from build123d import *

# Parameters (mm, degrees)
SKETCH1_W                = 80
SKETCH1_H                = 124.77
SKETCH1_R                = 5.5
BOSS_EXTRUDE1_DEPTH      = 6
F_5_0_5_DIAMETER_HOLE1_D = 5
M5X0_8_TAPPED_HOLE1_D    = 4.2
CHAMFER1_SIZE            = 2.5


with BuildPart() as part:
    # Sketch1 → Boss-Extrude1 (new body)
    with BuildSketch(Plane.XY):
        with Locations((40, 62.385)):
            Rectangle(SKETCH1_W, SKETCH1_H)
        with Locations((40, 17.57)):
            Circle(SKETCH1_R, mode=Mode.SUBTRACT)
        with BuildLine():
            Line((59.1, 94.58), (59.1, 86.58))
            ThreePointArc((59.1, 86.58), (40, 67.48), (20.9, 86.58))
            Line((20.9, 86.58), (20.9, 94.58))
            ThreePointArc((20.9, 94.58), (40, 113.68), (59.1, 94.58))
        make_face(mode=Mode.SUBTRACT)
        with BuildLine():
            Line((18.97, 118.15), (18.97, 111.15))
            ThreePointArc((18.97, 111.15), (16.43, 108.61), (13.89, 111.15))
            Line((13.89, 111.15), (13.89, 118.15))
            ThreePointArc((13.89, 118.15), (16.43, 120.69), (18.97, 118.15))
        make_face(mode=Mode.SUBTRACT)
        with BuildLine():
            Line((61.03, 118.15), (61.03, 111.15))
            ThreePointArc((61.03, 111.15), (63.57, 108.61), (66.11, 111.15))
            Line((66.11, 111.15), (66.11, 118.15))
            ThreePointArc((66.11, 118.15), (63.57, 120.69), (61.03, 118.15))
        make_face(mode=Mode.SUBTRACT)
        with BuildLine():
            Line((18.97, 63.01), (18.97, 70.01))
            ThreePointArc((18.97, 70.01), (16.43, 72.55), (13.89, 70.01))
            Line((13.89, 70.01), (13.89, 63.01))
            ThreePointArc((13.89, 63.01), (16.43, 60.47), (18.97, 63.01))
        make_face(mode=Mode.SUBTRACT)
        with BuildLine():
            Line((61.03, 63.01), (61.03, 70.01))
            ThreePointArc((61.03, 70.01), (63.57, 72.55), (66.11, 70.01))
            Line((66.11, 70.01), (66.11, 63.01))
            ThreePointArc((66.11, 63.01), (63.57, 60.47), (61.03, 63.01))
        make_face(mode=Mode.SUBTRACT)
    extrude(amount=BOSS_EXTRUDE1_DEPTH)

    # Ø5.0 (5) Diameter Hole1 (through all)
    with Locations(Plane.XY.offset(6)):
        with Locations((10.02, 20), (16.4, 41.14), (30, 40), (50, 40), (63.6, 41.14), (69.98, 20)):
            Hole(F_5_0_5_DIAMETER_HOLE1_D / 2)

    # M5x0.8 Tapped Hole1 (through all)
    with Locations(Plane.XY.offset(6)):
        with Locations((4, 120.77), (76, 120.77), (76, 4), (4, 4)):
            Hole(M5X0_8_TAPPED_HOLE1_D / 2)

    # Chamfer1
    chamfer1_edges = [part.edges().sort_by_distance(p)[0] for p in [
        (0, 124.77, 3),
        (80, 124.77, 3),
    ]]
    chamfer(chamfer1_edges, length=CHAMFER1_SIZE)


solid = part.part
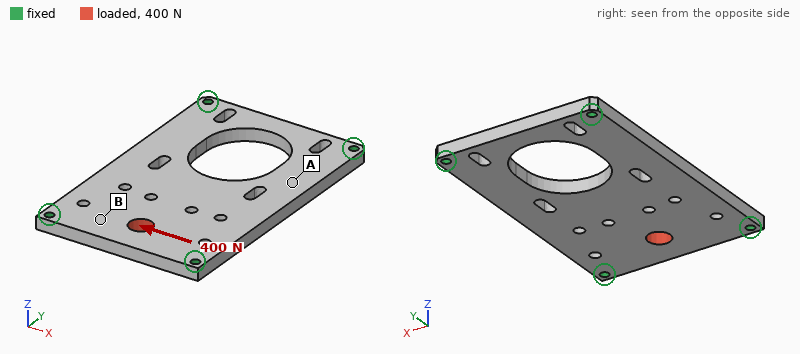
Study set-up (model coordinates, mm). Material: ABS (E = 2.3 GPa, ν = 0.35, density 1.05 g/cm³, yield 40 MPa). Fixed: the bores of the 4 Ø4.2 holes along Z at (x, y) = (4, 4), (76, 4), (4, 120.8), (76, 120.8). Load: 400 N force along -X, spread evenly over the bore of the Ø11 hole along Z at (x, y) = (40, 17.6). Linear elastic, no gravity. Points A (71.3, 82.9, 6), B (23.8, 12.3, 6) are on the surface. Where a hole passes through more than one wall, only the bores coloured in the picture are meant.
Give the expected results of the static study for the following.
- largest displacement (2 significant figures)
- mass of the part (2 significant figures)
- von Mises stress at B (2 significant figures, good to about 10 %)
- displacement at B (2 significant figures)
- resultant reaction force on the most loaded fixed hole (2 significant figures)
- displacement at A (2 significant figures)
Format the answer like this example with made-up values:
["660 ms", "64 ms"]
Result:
["38 µm", "51 g", "1.7 MPa", "22 µm", "190 N", "16 µm"]
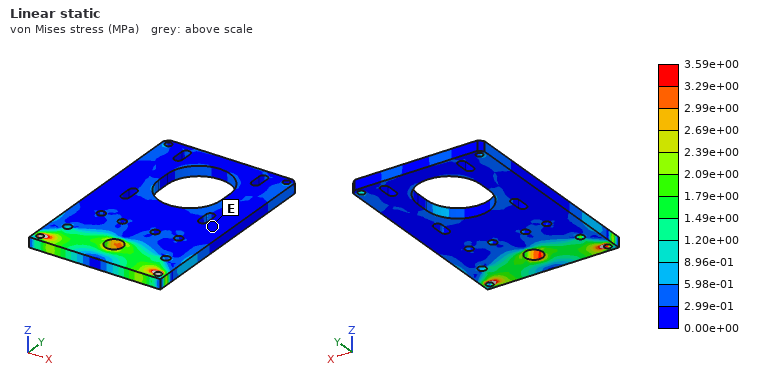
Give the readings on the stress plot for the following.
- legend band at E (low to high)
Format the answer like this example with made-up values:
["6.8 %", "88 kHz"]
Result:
["0.00e+00 to 2.99e-01 MPa"]
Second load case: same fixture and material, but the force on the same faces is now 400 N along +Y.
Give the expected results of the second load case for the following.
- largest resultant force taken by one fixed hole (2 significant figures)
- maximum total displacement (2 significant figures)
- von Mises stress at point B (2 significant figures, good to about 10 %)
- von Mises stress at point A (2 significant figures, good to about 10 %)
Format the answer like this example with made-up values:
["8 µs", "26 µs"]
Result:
["150 N", "53 µm", "1.1 MPa", "0.42 MPa"]
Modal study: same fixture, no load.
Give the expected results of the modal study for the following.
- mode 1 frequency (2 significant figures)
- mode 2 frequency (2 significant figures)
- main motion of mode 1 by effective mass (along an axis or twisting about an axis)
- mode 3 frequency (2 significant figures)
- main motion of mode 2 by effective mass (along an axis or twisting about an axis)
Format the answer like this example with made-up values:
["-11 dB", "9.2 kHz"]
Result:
["510 Hz", "810 Hz", "along Z", "1300 Hz", "twisting about Y"]
